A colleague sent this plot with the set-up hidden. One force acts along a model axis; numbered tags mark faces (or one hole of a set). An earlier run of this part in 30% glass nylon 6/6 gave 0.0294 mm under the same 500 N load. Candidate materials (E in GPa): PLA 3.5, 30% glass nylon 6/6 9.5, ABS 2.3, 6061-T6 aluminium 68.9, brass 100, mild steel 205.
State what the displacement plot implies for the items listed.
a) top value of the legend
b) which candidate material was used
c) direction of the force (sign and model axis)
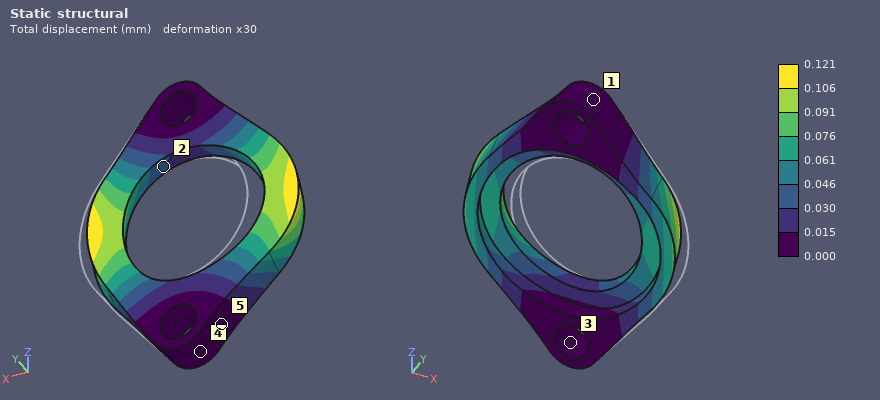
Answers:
0.121 mm
ABS
-X
